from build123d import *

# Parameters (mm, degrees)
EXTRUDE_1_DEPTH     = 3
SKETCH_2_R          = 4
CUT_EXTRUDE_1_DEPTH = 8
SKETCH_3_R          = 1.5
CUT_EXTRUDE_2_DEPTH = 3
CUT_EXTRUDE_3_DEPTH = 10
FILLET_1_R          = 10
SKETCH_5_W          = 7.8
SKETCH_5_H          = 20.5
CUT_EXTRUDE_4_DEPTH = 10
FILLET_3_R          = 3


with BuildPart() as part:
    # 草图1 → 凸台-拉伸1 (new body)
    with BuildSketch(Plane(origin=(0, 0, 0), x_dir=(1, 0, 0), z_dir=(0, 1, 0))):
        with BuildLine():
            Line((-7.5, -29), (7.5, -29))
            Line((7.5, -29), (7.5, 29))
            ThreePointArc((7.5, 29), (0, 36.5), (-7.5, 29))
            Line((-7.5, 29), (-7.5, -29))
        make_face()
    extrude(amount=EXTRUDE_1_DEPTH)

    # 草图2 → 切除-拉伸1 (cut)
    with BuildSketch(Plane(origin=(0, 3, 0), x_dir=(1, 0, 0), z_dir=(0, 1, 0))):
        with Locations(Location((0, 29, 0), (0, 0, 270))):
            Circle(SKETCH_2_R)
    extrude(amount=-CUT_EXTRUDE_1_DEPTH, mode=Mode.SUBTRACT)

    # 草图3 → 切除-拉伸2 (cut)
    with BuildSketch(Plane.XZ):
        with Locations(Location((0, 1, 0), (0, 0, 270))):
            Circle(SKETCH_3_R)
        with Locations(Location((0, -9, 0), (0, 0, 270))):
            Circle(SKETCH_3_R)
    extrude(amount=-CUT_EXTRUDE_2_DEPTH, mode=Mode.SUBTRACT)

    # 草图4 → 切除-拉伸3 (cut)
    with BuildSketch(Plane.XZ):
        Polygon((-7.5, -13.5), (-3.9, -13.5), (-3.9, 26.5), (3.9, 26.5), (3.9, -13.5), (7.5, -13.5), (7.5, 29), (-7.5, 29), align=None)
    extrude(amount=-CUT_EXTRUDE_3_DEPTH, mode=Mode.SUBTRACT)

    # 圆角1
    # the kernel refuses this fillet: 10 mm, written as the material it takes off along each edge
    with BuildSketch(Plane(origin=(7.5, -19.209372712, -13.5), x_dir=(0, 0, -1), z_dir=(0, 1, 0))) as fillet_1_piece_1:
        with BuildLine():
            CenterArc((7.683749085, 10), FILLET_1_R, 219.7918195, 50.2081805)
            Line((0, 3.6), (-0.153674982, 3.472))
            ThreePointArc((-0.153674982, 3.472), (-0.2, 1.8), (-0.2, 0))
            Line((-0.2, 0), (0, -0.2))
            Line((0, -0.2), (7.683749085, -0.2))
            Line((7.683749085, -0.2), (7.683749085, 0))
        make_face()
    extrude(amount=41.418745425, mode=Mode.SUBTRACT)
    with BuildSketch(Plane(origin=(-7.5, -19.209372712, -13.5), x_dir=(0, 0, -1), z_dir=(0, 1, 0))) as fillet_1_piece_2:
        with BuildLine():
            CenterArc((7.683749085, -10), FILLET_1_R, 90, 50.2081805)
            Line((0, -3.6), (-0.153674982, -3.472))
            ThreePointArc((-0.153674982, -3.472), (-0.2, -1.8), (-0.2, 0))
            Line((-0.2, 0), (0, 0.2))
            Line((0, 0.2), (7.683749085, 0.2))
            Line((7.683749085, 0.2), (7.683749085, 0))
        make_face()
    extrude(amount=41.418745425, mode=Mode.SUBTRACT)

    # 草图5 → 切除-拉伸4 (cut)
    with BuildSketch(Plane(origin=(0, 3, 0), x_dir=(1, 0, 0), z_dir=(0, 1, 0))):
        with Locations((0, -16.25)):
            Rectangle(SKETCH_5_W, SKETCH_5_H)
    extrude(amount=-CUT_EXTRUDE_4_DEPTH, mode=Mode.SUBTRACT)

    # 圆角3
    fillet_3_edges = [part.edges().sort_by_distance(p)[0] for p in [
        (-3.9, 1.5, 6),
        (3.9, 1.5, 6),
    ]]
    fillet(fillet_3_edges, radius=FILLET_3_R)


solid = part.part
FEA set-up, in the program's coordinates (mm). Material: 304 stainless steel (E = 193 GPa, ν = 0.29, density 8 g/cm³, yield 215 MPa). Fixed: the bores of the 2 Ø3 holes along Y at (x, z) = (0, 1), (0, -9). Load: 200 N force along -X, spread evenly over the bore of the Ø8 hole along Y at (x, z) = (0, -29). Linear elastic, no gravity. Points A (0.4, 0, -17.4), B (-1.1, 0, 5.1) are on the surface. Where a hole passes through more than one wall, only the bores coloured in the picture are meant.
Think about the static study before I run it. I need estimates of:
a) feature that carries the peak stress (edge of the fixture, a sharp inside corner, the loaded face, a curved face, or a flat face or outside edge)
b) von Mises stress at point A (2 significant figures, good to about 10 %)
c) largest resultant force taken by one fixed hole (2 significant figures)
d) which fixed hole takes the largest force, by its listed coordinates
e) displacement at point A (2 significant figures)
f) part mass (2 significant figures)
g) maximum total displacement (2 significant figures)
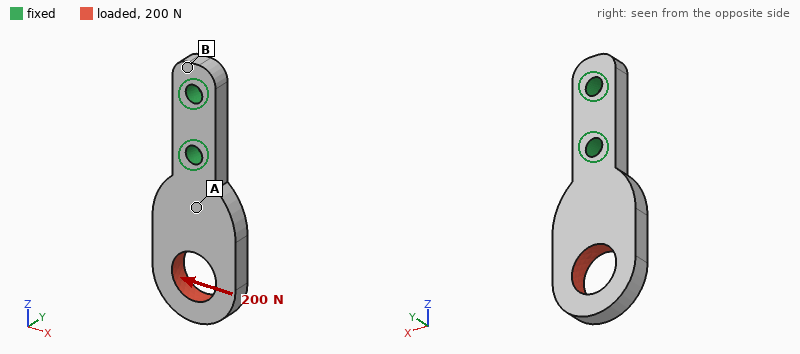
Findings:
edge of the fixture
31 MPa
340 N
(0, -9)
8.2 µm
9.3 g
37 µm
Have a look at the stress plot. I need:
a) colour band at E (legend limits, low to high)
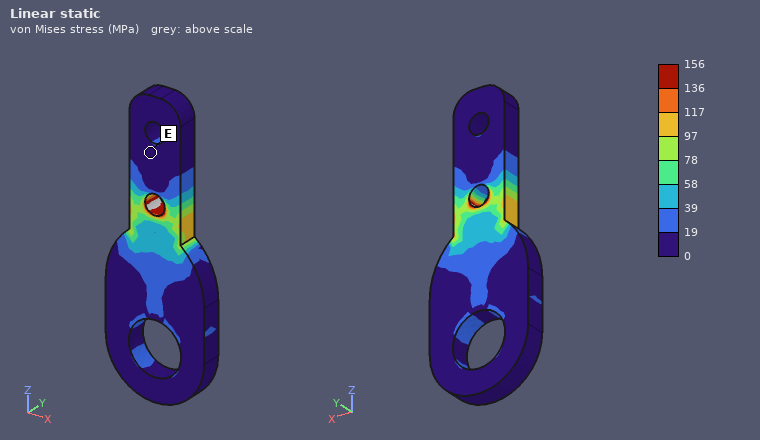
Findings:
0 to 19 MPa
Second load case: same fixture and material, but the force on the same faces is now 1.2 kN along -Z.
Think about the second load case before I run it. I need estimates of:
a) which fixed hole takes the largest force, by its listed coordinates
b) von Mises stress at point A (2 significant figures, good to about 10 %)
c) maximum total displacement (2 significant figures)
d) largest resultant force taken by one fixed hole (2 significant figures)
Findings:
(0, -9)
35 MPa
6.7 µm
1.1 kN
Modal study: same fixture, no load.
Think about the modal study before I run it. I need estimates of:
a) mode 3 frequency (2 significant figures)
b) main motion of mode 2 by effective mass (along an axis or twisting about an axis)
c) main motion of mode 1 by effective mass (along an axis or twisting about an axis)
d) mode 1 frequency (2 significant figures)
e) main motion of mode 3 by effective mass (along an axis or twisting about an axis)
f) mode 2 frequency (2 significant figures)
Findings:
9900 Hz
along X
along Y
3300 Hz
twisting about Z
6900 Hz
